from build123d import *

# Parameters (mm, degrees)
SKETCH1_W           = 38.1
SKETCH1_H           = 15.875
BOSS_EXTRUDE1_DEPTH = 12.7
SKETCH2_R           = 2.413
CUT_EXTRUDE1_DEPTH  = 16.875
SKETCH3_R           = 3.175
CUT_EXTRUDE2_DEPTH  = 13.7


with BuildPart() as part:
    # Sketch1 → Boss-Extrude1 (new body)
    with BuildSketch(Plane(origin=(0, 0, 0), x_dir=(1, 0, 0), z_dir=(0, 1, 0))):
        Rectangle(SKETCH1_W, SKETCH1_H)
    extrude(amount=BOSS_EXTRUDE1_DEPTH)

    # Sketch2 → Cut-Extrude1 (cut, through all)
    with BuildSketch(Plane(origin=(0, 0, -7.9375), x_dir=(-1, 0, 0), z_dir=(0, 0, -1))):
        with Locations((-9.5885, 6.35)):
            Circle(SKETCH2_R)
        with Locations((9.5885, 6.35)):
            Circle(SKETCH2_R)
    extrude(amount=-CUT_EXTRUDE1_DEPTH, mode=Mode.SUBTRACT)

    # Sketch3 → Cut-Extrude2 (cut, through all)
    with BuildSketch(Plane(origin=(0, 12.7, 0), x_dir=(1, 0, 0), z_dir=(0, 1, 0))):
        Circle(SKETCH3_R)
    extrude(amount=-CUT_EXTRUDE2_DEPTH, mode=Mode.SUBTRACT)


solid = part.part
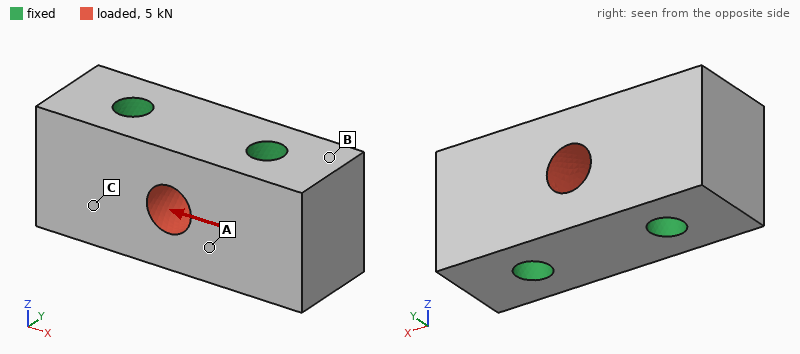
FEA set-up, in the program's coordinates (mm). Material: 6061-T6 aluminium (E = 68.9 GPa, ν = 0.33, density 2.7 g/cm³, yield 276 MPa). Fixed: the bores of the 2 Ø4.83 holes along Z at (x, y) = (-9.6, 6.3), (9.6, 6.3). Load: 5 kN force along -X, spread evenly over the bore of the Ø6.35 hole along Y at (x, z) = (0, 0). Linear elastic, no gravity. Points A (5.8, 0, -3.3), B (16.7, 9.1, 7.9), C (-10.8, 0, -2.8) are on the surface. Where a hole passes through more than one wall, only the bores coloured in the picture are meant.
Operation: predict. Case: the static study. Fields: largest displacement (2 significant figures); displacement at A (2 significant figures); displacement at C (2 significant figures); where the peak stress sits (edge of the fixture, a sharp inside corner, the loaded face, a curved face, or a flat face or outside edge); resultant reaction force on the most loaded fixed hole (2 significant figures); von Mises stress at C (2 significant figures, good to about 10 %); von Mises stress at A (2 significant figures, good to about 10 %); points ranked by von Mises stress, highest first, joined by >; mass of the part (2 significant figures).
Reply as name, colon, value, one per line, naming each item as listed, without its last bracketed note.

largest displacement: 2.2 µm
displacement at A: 1.2 µm
displacement at C: 0.52 µm
where the peak stress sits: the loaded face
resultant reaction force on the most loaded fixed hole: 2.5 kN
von Mises stress at C: 6.5 MPa
von Mises stress at A: 13 MPa
points ranked by von Mises stress, highest first, joined by >: A > C > B
mass of the part: 18 g
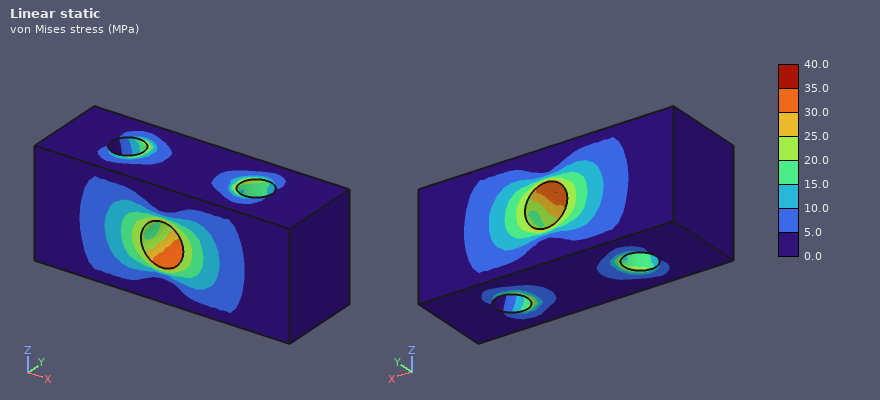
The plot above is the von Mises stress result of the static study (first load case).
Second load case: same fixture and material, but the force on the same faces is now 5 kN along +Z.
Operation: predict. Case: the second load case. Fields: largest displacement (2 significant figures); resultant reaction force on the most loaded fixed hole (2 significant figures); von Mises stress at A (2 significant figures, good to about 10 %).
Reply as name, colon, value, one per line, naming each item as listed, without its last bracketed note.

largest displacement: 5.0 µm
resultant reaction force on the most loaded fixed hole: 2.5 kN
von Mises stress at A: 19 MPa
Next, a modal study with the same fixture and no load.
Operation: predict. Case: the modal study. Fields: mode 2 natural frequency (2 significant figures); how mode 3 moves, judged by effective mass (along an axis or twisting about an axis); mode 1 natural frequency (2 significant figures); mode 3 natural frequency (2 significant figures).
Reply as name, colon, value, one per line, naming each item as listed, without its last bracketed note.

mode 2 natural frequency: 56 kHz
how mode 3 moves, judged by effective mass: twisting about Y
mode 1 natural frequency: 54 kHz
mode 3 natural frequency: 74 kHz
